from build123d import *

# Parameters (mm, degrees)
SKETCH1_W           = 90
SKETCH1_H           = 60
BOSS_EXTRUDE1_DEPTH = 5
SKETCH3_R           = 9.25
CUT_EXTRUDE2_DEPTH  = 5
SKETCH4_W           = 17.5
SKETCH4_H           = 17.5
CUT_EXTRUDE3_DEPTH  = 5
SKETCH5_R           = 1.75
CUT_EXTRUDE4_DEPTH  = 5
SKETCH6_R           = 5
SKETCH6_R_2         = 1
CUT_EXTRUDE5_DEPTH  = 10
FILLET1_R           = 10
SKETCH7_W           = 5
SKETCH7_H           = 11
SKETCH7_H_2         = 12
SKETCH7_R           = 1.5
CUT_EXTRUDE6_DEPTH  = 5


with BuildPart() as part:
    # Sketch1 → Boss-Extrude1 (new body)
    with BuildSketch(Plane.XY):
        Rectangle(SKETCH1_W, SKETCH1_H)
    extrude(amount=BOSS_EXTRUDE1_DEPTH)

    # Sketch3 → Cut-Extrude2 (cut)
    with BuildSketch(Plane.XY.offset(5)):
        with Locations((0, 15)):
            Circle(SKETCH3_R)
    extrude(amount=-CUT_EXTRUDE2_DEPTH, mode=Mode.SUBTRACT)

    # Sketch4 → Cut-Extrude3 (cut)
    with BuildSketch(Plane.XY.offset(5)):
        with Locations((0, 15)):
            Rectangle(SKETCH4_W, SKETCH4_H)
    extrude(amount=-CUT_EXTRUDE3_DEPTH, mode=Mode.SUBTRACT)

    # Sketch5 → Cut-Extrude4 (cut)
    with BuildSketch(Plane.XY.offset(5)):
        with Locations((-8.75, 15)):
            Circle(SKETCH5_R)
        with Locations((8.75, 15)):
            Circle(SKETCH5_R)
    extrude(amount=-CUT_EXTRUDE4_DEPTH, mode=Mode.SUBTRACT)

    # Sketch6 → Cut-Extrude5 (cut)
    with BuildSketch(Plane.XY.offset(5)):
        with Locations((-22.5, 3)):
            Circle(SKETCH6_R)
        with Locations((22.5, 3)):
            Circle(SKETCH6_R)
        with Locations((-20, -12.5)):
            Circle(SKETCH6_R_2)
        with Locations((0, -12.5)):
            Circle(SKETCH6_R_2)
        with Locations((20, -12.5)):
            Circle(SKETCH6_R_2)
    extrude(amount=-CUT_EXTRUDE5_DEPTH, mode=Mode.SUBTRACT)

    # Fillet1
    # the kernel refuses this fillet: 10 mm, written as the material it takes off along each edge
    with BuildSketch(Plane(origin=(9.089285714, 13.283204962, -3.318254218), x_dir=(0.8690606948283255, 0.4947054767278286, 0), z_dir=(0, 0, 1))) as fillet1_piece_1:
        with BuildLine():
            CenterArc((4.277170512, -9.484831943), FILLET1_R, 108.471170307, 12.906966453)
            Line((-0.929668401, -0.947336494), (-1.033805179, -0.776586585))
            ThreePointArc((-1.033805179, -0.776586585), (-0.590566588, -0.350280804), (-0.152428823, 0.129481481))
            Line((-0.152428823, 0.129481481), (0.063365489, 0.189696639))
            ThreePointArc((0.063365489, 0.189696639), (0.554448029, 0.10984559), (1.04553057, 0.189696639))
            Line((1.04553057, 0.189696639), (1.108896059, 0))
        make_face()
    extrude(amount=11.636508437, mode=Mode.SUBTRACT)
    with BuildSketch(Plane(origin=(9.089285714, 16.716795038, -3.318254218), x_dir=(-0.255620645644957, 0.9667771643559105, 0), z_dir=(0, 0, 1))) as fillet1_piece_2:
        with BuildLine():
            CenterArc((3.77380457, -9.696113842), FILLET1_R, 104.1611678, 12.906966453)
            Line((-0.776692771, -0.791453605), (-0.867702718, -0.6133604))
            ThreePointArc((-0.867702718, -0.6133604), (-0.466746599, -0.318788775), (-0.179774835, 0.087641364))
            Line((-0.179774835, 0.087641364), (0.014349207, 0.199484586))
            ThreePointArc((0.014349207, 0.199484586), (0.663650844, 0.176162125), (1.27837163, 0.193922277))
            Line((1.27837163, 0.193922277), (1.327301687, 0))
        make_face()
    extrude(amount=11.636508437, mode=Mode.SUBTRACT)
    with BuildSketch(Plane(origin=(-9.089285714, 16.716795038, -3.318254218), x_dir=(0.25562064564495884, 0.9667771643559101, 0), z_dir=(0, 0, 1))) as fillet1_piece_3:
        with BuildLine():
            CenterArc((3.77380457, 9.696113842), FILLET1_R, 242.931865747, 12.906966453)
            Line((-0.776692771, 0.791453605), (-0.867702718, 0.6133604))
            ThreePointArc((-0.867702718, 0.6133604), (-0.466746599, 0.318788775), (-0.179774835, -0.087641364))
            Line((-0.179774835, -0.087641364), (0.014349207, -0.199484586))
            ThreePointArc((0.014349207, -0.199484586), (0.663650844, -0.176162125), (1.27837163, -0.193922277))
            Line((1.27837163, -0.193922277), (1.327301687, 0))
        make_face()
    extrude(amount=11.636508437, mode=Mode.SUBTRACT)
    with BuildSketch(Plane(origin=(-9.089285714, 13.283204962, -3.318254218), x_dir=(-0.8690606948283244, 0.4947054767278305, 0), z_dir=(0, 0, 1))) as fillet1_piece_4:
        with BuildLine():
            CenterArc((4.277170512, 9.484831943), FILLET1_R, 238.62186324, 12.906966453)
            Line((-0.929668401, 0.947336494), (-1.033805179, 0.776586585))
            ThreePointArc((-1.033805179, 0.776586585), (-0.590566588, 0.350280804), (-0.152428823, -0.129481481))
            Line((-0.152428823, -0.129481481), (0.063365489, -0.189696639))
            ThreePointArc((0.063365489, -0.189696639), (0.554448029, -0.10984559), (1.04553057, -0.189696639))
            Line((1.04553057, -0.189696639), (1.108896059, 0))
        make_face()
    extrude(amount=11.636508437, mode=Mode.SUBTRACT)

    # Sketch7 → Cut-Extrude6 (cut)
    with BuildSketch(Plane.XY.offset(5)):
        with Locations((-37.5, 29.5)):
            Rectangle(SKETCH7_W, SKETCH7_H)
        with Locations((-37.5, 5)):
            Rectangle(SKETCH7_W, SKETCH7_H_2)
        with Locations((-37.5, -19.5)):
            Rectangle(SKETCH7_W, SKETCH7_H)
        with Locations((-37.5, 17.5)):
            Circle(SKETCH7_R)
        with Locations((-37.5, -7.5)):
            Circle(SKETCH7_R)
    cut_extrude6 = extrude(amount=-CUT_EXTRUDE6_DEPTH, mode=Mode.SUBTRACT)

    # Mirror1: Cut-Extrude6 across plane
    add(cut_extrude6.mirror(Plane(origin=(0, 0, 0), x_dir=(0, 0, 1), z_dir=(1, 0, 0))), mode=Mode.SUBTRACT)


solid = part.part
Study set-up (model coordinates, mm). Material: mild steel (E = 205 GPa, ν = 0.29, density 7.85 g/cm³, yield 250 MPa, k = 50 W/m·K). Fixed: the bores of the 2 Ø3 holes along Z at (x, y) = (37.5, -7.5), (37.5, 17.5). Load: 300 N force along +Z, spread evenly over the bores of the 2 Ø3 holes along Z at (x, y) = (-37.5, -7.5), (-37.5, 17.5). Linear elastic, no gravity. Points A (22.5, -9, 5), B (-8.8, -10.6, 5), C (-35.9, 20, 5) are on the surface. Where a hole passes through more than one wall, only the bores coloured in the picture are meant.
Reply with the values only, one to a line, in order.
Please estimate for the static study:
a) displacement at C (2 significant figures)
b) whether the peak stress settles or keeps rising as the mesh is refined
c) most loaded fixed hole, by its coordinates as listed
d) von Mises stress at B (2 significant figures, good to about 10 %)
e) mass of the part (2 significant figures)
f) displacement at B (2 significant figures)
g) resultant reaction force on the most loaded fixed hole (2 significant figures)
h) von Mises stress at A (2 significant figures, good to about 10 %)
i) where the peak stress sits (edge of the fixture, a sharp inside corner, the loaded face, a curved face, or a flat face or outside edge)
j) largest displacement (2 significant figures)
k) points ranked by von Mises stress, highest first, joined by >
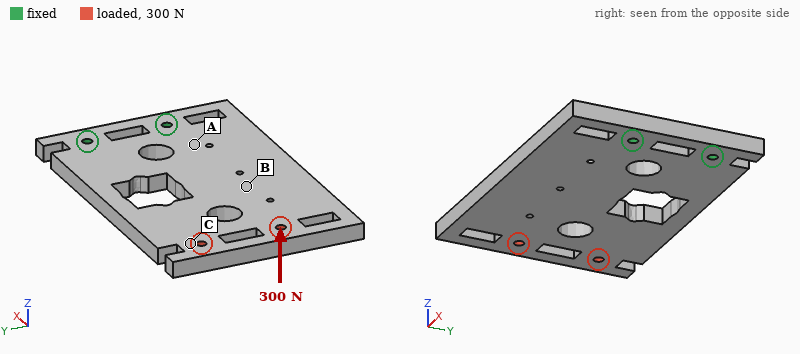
0.49 mm
keeps rising
(37.5, -7.5)
46 MPa
180 g
0.24 mm
160 N
93 MPa
edge of the fixture
0.58 mm
A > B > C
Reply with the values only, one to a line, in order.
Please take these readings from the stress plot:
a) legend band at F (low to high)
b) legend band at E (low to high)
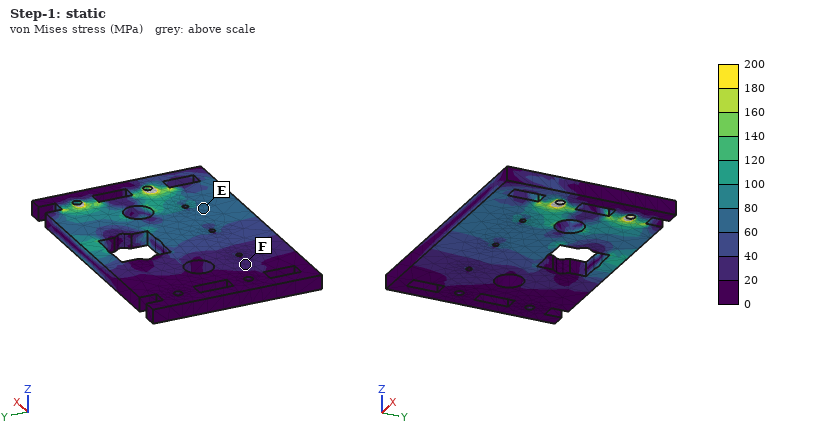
20 to 40 MPa
60 to 80 MPa
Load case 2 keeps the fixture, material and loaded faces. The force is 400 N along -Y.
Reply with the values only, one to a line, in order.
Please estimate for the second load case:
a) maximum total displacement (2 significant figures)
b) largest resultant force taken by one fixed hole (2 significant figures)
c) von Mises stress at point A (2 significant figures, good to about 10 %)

18 µm
1.1 kN
9.9 MPa
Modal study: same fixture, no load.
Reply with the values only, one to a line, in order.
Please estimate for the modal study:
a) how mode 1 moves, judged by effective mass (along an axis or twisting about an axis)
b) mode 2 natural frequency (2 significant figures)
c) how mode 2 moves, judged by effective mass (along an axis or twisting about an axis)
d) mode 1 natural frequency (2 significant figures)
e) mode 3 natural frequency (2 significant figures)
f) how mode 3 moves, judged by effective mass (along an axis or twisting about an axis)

along Z
1600 Hz
twisting about X
530 Hz
3100 Hz
along Y
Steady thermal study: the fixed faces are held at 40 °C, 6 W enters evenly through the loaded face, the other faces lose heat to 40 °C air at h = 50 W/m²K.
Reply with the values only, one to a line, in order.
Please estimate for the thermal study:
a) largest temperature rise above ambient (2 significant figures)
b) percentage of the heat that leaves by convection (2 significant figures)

22 K
77 %
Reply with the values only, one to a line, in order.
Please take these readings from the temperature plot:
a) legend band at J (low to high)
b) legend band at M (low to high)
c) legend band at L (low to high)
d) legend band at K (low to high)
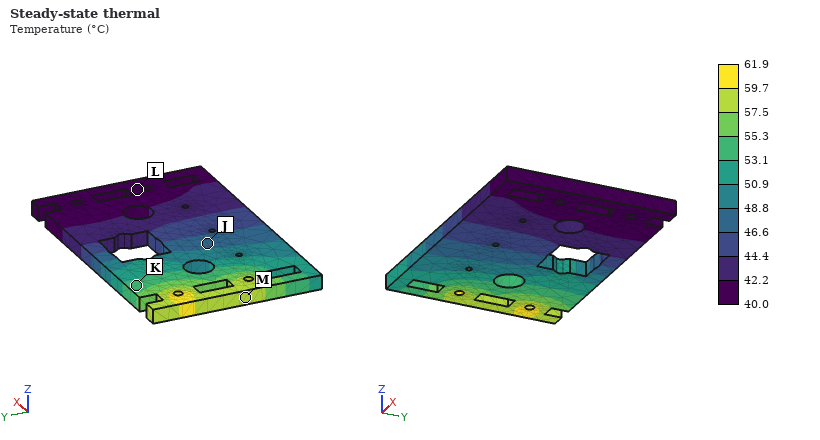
46.6 to 48.8 °C
57.5 to 59.7 °C
40.0 to 42.2 °C
53.1 to 55.3 °C
